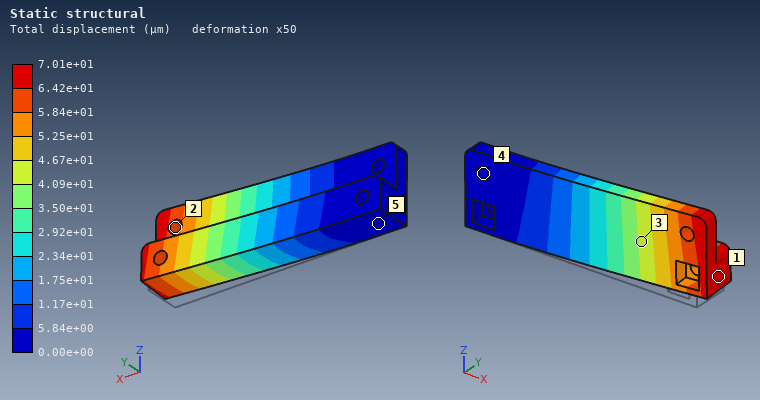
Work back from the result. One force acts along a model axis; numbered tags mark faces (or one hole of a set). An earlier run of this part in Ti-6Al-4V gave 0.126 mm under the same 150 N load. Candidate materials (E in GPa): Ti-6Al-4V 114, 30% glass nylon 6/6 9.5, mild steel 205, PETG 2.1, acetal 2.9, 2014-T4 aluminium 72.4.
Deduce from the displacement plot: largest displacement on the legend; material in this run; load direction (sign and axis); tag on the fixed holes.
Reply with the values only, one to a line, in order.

7.01e+01 µm
mild steel
+Y
4
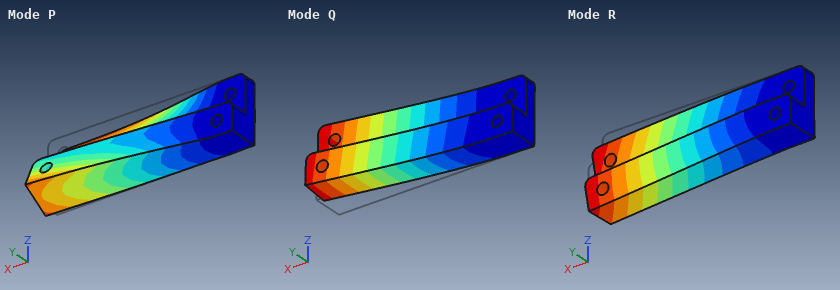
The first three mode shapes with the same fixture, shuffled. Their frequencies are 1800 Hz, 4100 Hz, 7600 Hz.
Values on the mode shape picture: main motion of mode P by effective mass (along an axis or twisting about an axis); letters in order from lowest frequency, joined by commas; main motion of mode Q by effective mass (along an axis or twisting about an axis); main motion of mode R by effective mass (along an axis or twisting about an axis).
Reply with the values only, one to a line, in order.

twisting about X
Q, R, P
along Y
along Z
